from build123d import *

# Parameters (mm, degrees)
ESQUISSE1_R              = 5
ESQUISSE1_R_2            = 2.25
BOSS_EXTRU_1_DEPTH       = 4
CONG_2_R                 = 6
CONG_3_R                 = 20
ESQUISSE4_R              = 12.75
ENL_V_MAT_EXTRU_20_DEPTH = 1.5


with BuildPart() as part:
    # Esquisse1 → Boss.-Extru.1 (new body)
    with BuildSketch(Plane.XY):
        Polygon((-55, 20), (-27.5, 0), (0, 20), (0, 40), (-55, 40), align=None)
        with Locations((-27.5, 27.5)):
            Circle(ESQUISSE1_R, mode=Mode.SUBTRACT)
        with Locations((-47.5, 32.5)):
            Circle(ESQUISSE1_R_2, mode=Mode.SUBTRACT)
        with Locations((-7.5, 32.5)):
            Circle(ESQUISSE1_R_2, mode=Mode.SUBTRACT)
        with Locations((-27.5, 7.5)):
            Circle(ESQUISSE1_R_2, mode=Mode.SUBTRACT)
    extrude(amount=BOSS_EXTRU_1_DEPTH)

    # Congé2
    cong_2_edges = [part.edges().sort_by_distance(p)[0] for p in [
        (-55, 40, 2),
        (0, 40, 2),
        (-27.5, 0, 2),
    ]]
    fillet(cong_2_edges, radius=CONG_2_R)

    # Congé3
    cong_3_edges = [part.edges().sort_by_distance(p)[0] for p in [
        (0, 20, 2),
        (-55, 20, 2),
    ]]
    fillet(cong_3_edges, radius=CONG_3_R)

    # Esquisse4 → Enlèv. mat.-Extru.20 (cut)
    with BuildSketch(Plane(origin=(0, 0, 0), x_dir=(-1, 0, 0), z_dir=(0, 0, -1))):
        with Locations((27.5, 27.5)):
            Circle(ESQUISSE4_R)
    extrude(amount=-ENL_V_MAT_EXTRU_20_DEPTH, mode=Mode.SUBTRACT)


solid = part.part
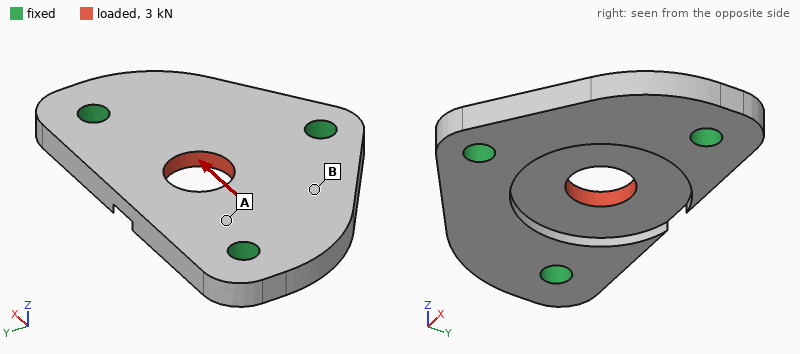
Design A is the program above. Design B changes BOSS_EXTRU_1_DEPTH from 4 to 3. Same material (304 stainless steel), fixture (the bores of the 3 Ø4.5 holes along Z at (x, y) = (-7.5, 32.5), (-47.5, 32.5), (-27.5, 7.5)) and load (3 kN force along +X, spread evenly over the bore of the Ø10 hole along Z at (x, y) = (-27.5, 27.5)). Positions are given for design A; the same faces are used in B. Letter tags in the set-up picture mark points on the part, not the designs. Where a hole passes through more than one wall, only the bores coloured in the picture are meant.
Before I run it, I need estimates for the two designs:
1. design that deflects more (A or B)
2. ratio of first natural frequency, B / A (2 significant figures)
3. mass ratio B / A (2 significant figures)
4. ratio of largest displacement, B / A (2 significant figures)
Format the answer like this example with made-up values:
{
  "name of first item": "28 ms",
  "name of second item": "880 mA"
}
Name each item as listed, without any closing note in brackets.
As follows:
{
  "design that deflects more": "B",
  "ratio of first natural frequency, B / A": "0.80",
  "mass ratio B / A": "0.72",
  "ratio of largest displacement, B / A": "1.6"
}
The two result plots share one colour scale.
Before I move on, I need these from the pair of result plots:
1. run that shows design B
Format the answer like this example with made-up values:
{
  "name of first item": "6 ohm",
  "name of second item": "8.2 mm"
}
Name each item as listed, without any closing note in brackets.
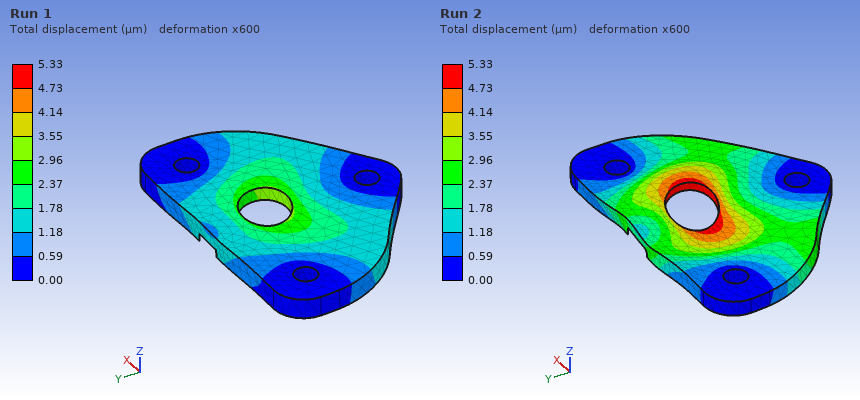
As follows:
{
  "run that shows design B": "Run 2"
}
